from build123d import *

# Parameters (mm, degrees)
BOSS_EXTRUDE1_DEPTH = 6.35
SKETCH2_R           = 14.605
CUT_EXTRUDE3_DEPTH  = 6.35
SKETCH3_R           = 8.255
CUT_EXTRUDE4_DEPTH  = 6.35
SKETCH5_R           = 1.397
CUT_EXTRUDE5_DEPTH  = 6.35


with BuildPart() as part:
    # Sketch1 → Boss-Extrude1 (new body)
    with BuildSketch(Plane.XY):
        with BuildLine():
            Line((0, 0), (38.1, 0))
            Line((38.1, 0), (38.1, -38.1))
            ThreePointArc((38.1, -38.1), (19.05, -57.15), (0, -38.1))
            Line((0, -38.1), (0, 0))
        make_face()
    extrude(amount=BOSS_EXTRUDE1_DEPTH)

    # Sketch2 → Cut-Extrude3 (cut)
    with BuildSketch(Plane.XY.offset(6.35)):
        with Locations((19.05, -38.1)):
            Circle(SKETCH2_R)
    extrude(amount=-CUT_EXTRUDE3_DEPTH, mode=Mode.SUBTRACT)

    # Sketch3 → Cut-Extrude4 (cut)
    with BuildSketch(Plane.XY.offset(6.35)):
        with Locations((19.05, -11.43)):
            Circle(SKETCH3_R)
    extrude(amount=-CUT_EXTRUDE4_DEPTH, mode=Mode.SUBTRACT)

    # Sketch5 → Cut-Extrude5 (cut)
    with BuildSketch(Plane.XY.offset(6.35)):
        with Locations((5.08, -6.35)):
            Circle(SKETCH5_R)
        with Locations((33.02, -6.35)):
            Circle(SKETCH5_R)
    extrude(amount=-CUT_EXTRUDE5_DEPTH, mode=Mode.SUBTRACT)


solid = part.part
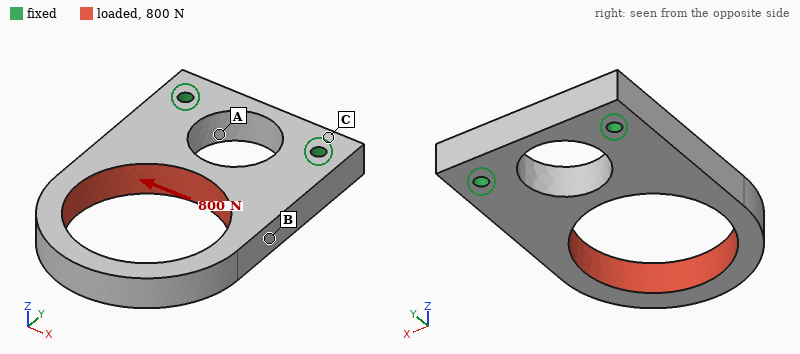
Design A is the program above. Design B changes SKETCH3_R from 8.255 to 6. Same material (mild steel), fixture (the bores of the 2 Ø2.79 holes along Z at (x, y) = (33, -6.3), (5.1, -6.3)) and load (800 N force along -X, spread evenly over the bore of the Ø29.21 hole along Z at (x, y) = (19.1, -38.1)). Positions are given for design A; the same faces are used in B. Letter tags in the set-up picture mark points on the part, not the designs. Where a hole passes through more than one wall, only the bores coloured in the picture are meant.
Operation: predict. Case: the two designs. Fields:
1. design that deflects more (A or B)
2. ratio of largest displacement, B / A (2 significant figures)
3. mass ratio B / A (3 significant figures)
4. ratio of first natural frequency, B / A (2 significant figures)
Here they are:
A
0.83
1.09
1.0
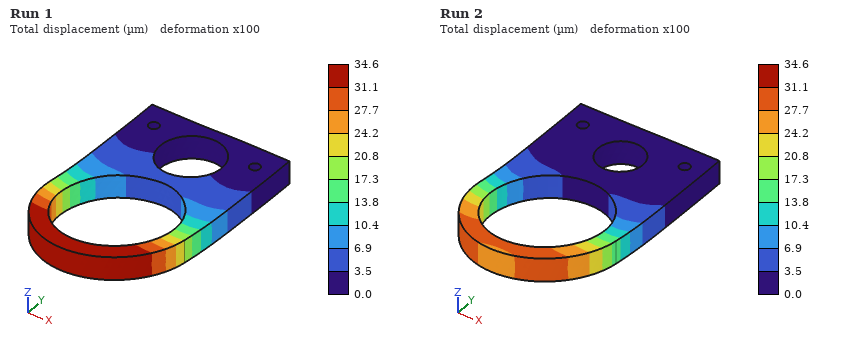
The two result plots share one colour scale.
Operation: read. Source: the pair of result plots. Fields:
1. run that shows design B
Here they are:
Run 2
